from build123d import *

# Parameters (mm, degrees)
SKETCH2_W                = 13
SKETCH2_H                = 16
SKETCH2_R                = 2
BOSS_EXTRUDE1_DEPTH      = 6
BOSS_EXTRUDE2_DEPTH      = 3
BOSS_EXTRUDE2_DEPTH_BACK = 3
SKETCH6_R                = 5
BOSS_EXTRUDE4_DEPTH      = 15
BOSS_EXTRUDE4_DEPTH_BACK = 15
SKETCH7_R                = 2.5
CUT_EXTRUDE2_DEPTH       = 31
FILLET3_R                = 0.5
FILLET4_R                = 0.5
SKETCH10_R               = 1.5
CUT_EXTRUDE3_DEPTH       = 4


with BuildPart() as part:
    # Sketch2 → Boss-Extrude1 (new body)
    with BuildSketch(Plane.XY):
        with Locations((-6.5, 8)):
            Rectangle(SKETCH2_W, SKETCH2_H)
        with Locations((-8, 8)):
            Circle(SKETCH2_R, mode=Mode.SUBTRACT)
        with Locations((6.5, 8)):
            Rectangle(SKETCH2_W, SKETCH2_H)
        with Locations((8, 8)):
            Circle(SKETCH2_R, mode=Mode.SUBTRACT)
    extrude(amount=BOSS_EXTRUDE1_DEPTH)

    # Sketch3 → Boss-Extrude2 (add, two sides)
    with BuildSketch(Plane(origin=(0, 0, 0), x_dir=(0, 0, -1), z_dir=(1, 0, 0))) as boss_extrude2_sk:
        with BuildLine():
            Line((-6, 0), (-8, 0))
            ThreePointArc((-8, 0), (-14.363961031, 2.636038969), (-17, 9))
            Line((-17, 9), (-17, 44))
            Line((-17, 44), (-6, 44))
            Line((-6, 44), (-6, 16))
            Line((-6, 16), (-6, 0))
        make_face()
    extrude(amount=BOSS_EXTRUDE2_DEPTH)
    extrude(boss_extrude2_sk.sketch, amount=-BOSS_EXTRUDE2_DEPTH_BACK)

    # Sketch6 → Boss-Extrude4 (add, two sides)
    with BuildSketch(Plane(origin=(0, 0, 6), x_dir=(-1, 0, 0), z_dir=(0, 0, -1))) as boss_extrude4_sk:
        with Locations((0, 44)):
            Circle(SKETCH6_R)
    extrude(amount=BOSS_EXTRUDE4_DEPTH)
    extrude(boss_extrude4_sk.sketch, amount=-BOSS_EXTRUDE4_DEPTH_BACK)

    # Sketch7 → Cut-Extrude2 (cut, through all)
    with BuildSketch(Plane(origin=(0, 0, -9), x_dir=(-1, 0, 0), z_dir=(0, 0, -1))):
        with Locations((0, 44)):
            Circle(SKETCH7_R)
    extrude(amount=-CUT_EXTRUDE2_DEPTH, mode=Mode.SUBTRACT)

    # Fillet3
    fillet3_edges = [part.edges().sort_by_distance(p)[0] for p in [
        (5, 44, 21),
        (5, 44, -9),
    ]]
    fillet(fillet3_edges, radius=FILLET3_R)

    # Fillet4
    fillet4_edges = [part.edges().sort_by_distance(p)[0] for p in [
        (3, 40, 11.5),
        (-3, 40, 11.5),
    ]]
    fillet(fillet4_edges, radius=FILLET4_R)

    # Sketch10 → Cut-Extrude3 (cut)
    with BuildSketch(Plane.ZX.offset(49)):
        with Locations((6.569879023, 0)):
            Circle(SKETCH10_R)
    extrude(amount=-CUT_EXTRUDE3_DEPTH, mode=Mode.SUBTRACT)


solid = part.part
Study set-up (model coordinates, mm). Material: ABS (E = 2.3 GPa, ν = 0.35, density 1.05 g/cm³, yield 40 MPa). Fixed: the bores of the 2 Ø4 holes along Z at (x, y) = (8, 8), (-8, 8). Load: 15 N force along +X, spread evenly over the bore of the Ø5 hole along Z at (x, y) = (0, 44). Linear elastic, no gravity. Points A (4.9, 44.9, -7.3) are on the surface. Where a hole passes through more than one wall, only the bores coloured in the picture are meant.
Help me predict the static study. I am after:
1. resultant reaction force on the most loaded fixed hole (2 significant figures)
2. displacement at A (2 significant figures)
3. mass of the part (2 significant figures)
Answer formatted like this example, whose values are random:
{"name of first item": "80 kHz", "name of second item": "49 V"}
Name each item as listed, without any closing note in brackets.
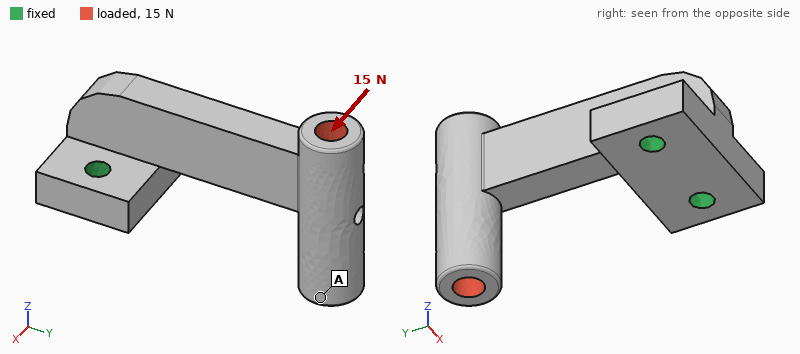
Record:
{"resultant reaction force on the most loaded fixed hole": "31 N", "displacement at A": "0.52 mm", "mass of the part": "6.9 g"}
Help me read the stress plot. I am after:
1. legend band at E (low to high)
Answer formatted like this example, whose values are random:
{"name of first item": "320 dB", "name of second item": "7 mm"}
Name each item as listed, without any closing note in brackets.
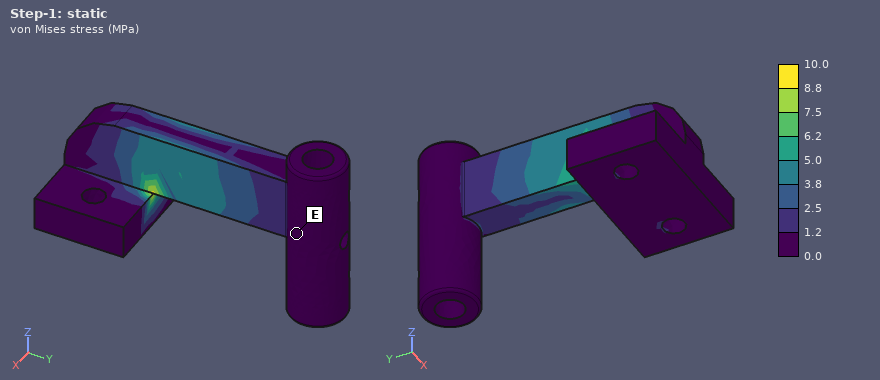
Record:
{"legend band at E": "0.0 to 1.2 MPa"}
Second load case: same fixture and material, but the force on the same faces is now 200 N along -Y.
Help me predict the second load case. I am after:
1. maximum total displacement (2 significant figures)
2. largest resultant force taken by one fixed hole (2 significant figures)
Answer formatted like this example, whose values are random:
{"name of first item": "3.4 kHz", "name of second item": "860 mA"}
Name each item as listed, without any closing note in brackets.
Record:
{"maximum total displacement": "0.71 mm", "largest resultant force taken by one fixed hole": "100 N"}
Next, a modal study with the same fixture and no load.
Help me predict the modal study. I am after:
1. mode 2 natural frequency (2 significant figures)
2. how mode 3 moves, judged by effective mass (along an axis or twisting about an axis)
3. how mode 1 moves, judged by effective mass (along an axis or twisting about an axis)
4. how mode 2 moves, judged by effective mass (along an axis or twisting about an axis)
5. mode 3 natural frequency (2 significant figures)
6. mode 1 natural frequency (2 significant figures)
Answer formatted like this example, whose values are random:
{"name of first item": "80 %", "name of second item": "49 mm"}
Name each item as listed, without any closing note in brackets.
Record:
{"mode 2 natural frequency": "880 Hz", "how mode 3 moves, judged by effective mass": "twisting about Y", "how mode 1 moves, judged by effective mass": "along X", "how mode 2 moves, judged by effective mass": "along Z", "mode 3 natural frequency": "1400 Hz", "mode 1 natural frequency": "640 Hz"}
